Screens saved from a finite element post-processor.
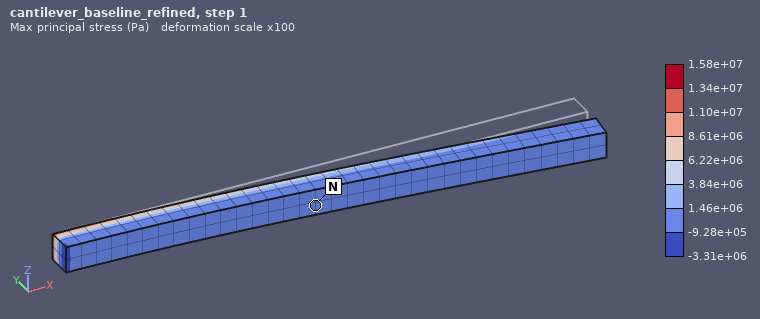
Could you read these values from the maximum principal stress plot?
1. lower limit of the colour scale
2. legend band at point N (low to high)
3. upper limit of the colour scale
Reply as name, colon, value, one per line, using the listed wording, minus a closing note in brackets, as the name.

lower limit of the colour scale: -3.31e+06 Pa
legend band at point N: -9.28e+05 to 1.46e+06 Pa
upper limit of the colour scale: 1.58e+07 Pa
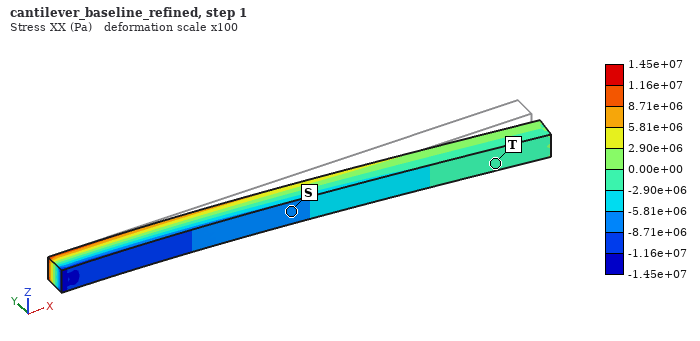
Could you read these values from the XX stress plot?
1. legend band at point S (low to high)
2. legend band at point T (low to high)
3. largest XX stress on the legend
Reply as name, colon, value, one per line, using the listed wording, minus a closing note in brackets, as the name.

legend band at point S: -8.71e+06 to -5.81e+06 Pa
legend band at point T: -2.90e+06 to 0.00e+00 Pa
largest XX stress on the legend: 1.45e+07 Pa
